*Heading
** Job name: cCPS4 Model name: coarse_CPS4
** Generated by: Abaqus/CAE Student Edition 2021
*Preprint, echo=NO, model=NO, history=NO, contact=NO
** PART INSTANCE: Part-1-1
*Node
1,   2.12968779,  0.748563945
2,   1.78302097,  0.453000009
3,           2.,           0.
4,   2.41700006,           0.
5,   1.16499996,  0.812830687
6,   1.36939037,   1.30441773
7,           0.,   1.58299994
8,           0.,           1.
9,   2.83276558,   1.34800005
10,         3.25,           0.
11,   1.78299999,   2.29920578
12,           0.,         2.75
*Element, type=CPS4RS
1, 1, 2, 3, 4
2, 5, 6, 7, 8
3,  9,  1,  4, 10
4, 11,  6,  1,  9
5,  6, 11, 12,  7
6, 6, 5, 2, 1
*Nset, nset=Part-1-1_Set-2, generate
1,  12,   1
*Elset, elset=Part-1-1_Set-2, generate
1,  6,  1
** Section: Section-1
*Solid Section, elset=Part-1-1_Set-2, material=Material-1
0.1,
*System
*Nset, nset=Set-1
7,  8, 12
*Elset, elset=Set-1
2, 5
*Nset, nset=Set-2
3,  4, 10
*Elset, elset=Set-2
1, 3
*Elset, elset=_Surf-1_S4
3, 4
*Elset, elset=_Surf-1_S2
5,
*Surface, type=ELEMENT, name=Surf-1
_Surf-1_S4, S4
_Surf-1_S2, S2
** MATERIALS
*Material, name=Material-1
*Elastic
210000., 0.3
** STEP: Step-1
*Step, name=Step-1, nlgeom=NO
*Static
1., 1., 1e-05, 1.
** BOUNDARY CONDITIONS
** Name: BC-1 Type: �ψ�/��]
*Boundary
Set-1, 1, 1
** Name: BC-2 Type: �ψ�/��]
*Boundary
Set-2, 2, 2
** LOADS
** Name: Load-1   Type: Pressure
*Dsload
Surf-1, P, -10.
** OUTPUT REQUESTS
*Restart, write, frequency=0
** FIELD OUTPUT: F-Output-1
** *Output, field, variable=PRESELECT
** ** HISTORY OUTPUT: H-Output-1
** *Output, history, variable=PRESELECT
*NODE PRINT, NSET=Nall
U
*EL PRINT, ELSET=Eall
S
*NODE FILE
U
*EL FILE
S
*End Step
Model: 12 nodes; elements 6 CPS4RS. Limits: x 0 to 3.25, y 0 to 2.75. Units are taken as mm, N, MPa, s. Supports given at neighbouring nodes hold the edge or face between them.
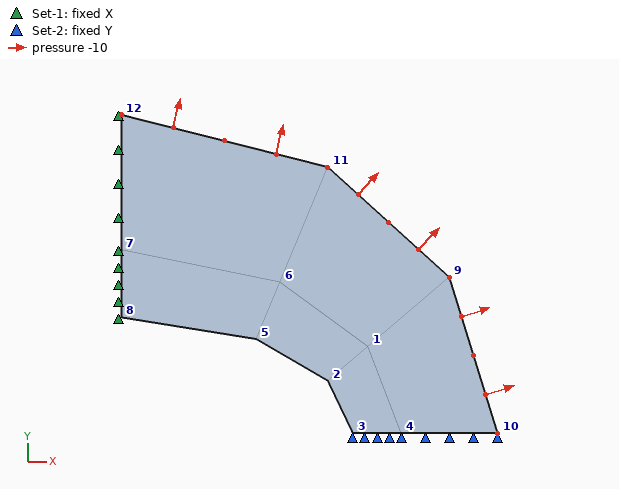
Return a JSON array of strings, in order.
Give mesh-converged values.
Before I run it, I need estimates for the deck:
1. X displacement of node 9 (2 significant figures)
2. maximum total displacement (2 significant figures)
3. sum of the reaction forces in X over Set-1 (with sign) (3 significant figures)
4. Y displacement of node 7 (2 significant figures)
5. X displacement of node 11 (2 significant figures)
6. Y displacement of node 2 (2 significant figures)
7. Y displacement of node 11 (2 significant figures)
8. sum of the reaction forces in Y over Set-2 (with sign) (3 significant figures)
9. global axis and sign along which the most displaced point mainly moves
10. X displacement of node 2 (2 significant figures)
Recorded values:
["7.4e-05 mm", "5.6e-04 mm", "-2.75 N", "5.5e-04 mm", "1.9e-04 mm", "2.0e-04 mm", "3.2e-04 mm", "-3.25 N", "+Y", "-8.7e-05 mm"]
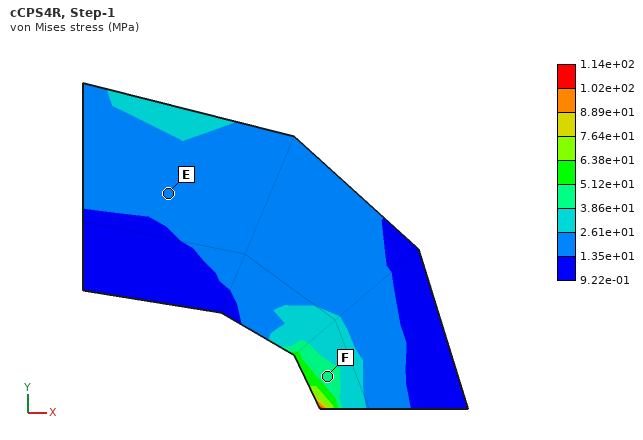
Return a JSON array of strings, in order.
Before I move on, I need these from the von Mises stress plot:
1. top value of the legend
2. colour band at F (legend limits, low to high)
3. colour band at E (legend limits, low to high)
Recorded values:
["1.14e+02 MPa", "3.86e+01 to 5.12e+01 MPa", "1.35e+01 to 2.61e+01 MPa"]
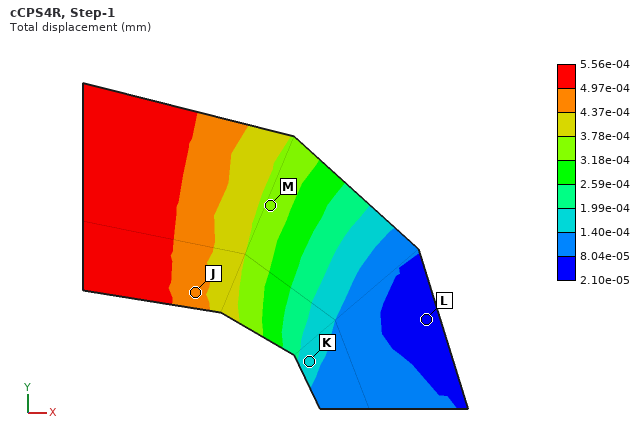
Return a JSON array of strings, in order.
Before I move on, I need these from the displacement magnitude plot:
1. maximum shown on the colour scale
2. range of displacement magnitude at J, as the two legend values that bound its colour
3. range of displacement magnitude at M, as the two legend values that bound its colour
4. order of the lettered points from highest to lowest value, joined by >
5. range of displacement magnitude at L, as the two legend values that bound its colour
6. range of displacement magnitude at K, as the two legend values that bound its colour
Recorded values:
["5.56e-04 mm", "4.37e-04 to 4.97e-04 mm", "3.18e-04 to 3.78e-04 mm", "J > M > K > L", "2.10e-05 to 8.04e-05 mm", "1.40e-04 to 1.99e-04 mm"]
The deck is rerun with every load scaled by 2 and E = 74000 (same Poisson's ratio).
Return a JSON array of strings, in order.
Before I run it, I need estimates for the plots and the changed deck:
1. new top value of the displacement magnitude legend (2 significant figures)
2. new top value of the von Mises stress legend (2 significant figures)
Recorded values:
["0.0032 mm", "230 MPa"]
